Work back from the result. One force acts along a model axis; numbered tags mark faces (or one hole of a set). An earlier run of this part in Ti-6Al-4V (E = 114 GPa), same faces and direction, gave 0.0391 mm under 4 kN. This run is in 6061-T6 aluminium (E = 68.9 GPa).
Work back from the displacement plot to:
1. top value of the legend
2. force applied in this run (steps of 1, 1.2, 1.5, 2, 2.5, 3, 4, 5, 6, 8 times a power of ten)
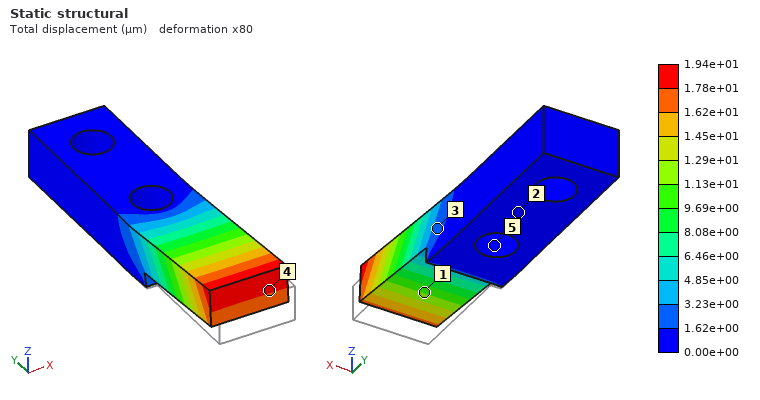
1.94e+01 µm
1.2 kN
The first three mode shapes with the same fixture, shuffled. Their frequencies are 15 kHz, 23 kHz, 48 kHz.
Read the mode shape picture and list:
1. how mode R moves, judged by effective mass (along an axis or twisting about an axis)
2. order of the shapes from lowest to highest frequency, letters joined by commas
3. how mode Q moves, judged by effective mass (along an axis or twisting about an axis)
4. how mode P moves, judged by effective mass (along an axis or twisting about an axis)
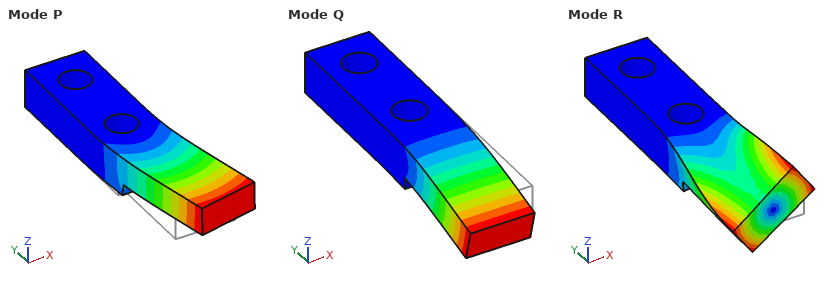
twisting about Y
Q, P, R
along Z
along X
